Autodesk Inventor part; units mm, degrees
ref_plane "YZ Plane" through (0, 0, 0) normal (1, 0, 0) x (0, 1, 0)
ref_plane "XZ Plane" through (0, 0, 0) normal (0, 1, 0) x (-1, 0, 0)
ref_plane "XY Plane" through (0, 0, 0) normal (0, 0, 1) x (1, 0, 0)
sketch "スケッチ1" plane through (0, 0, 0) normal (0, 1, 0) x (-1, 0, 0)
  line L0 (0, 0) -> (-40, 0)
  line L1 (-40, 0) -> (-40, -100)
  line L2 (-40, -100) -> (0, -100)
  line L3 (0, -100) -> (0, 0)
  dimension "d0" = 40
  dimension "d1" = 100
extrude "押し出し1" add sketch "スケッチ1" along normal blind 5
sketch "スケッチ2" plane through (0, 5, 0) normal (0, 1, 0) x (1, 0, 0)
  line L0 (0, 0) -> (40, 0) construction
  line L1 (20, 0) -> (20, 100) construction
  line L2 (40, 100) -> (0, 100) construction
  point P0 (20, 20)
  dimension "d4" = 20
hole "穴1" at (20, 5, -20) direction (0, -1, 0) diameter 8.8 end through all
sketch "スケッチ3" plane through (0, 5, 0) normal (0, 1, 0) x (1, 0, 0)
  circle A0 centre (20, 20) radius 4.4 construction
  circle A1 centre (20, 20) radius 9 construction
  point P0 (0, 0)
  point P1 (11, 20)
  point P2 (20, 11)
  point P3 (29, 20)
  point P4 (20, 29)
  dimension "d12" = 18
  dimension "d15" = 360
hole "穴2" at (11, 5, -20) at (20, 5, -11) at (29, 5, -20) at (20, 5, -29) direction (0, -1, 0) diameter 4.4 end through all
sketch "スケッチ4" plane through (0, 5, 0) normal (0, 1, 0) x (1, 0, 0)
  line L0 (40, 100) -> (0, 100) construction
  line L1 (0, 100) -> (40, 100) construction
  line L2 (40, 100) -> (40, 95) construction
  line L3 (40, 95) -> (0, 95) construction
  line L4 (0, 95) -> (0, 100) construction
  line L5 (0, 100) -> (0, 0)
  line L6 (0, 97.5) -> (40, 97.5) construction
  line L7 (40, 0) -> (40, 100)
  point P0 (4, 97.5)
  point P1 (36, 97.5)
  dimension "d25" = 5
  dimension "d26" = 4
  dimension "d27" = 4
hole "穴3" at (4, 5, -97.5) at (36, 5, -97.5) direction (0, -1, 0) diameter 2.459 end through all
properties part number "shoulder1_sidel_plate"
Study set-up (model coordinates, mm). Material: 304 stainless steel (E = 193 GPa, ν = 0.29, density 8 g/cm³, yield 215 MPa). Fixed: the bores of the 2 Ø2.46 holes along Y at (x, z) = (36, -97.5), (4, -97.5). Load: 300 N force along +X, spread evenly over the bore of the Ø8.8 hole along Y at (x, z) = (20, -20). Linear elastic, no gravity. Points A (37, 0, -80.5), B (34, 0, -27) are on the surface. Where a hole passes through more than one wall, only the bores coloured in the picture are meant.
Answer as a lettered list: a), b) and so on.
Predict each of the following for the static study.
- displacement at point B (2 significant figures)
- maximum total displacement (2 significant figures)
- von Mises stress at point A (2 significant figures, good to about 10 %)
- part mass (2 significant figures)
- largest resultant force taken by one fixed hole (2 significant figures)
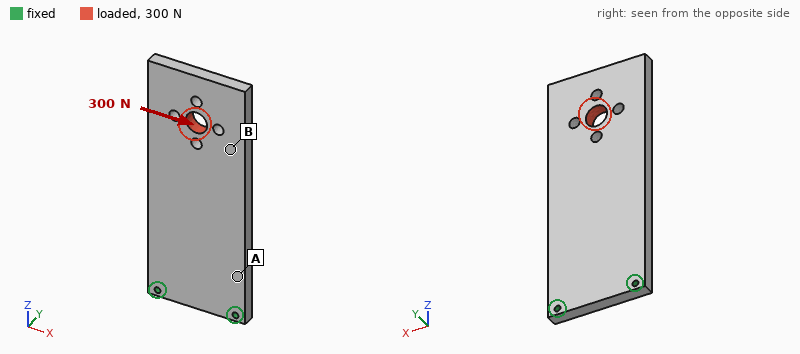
a) 11 µm
b) 16 µm
c) 12 MPa
d) 150 g
e) 730 N
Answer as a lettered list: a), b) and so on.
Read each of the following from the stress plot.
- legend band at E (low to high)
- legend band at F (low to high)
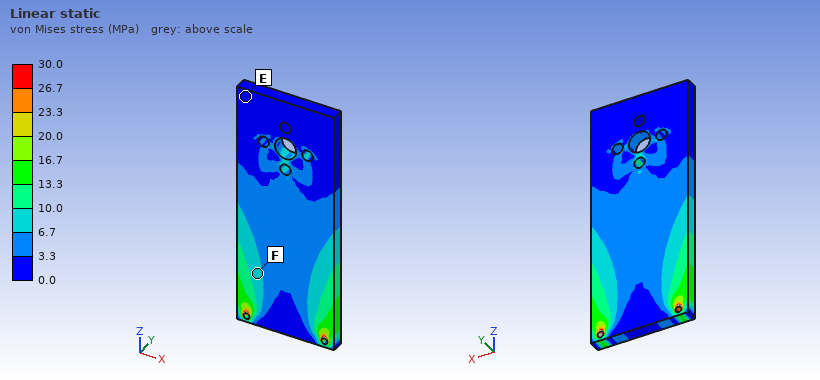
a) 0.0 to 3.3 MPa
b) 6.7 to 10.0 MPa
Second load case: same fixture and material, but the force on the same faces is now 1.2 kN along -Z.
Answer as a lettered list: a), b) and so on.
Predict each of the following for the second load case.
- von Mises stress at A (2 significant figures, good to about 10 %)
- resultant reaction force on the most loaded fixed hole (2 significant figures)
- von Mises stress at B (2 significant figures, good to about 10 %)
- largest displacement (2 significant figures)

a) 7.6 MPa
b) 620 N
c) 4.1 MPa
d) 3.8 µm
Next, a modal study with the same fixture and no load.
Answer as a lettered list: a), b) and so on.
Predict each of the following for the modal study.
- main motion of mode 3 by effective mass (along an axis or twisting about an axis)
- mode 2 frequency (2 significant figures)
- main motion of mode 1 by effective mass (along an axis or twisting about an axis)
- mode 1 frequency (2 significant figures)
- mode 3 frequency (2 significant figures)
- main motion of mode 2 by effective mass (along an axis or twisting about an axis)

a) along Y
b) 2100 Hz
c) along Y
d) 390 Hz
e) 2400 Hz
f) twisting about Z
